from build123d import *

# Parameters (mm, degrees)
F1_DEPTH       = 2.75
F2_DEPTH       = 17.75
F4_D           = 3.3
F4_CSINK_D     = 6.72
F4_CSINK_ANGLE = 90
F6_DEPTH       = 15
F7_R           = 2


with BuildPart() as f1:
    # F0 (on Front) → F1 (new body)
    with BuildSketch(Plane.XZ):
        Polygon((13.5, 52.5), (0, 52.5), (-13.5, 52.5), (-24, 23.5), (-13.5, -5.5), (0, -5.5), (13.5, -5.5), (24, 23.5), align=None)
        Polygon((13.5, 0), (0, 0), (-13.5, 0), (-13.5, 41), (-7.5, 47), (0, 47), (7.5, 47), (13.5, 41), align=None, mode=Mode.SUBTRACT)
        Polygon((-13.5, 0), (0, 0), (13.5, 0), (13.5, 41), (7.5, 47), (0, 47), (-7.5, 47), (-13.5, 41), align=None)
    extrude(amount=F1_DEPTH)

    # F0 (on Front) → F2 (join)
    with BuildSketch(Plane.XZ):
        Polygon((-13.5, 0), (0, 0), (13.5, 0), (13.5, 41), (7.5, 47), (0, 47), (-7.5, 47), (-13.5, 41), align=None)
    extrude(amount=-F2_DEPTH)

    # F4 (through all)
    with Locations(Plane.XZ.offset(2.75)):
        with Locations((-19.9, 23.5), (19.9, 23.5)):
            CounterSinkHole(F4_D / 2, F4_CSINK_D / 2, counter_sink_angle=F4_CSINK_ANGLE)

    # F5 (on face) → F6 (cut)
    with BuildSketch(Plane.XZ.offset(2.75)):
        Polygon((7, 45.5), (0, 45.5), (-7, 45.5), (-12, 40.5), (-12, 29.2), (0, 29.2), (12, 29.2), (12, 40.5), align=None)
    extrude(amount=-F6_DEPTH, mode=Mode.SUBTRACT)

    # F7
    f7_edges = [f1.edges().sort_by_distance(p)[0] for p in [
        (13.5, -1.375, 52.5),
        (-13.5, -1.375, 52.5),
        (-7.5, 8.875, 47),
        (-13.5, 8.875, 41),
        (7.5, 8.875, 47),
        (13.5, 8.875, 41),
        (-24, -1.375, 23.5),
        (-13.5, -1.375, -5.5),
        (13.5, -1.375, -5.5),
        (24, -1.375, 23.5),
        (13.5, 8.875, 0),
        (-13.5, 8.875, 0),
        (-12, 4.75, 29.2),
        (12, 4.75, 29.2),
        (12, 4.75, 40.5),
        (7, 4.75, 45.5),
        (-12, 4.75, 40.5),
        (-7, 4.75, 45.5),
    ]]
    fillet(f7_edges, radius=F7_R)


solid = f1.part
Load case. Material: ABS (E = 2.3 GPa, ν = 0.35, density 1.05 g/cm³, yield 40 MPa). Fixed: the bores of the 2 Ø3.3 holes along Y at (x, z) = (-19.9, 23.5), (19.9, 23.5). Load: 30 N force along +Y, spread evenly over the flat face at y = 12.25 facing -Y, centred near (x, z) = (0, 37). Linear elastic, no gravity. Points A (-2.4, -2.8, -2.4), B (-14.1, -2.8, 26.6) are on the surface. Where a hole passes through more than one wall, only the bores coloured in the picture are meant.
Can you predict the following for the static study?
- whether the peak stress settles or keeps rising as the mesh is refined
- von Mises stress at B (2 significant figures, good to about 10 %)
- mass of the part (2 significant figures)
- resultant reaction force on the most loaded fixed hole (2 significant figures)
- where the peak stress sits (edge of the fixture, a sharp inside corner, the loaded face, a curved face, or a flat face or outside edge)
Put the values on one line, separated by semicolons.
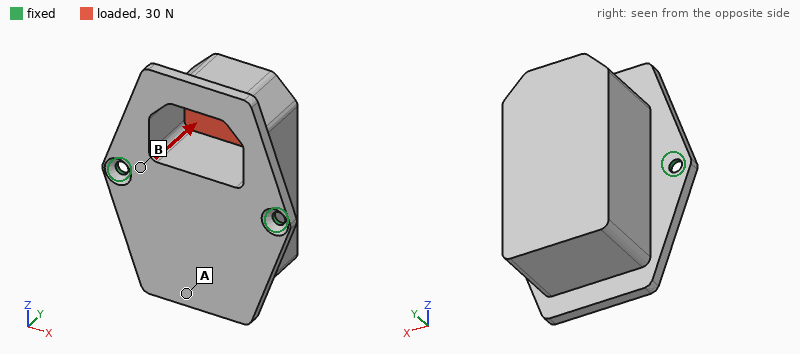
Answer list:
keeps rising; 5.9 MPa; 23 g; 15 N; edge of the fixture
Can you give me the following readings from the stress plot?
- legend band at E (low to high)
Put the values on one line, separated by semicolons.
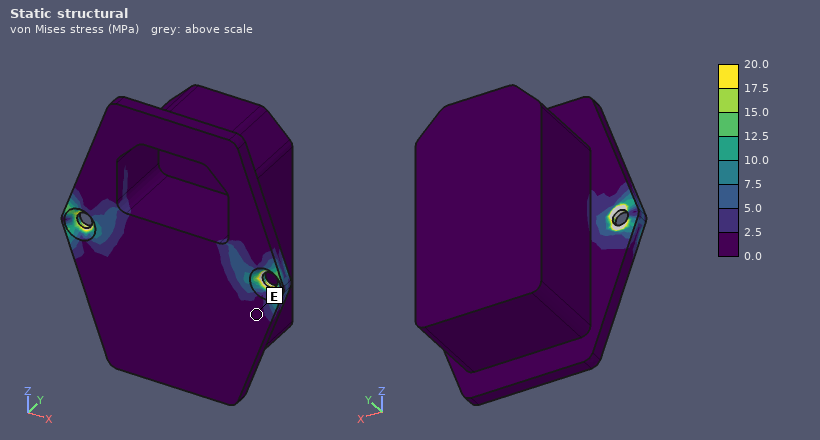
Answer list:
0.0 to 2.5 MPa
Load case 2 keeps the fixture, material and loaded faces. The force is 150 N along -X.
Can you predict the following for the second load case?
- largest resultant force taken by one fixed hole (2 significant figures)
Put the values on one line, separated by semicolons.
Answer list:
110 N
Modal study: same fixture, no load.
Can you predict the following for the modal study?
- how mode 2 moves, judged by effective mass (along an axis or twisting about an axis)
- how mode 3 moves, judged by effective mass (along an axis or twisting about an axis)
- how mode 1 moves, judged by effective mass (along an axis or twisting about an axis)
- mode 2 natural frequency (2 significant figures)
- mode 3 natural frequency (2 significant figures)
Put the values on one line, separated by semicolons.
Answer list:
along Y; along X; along Z; 1200 Hz; 1500 Hz
